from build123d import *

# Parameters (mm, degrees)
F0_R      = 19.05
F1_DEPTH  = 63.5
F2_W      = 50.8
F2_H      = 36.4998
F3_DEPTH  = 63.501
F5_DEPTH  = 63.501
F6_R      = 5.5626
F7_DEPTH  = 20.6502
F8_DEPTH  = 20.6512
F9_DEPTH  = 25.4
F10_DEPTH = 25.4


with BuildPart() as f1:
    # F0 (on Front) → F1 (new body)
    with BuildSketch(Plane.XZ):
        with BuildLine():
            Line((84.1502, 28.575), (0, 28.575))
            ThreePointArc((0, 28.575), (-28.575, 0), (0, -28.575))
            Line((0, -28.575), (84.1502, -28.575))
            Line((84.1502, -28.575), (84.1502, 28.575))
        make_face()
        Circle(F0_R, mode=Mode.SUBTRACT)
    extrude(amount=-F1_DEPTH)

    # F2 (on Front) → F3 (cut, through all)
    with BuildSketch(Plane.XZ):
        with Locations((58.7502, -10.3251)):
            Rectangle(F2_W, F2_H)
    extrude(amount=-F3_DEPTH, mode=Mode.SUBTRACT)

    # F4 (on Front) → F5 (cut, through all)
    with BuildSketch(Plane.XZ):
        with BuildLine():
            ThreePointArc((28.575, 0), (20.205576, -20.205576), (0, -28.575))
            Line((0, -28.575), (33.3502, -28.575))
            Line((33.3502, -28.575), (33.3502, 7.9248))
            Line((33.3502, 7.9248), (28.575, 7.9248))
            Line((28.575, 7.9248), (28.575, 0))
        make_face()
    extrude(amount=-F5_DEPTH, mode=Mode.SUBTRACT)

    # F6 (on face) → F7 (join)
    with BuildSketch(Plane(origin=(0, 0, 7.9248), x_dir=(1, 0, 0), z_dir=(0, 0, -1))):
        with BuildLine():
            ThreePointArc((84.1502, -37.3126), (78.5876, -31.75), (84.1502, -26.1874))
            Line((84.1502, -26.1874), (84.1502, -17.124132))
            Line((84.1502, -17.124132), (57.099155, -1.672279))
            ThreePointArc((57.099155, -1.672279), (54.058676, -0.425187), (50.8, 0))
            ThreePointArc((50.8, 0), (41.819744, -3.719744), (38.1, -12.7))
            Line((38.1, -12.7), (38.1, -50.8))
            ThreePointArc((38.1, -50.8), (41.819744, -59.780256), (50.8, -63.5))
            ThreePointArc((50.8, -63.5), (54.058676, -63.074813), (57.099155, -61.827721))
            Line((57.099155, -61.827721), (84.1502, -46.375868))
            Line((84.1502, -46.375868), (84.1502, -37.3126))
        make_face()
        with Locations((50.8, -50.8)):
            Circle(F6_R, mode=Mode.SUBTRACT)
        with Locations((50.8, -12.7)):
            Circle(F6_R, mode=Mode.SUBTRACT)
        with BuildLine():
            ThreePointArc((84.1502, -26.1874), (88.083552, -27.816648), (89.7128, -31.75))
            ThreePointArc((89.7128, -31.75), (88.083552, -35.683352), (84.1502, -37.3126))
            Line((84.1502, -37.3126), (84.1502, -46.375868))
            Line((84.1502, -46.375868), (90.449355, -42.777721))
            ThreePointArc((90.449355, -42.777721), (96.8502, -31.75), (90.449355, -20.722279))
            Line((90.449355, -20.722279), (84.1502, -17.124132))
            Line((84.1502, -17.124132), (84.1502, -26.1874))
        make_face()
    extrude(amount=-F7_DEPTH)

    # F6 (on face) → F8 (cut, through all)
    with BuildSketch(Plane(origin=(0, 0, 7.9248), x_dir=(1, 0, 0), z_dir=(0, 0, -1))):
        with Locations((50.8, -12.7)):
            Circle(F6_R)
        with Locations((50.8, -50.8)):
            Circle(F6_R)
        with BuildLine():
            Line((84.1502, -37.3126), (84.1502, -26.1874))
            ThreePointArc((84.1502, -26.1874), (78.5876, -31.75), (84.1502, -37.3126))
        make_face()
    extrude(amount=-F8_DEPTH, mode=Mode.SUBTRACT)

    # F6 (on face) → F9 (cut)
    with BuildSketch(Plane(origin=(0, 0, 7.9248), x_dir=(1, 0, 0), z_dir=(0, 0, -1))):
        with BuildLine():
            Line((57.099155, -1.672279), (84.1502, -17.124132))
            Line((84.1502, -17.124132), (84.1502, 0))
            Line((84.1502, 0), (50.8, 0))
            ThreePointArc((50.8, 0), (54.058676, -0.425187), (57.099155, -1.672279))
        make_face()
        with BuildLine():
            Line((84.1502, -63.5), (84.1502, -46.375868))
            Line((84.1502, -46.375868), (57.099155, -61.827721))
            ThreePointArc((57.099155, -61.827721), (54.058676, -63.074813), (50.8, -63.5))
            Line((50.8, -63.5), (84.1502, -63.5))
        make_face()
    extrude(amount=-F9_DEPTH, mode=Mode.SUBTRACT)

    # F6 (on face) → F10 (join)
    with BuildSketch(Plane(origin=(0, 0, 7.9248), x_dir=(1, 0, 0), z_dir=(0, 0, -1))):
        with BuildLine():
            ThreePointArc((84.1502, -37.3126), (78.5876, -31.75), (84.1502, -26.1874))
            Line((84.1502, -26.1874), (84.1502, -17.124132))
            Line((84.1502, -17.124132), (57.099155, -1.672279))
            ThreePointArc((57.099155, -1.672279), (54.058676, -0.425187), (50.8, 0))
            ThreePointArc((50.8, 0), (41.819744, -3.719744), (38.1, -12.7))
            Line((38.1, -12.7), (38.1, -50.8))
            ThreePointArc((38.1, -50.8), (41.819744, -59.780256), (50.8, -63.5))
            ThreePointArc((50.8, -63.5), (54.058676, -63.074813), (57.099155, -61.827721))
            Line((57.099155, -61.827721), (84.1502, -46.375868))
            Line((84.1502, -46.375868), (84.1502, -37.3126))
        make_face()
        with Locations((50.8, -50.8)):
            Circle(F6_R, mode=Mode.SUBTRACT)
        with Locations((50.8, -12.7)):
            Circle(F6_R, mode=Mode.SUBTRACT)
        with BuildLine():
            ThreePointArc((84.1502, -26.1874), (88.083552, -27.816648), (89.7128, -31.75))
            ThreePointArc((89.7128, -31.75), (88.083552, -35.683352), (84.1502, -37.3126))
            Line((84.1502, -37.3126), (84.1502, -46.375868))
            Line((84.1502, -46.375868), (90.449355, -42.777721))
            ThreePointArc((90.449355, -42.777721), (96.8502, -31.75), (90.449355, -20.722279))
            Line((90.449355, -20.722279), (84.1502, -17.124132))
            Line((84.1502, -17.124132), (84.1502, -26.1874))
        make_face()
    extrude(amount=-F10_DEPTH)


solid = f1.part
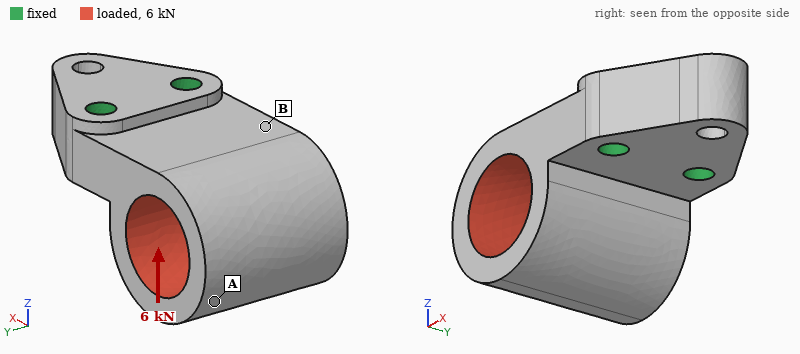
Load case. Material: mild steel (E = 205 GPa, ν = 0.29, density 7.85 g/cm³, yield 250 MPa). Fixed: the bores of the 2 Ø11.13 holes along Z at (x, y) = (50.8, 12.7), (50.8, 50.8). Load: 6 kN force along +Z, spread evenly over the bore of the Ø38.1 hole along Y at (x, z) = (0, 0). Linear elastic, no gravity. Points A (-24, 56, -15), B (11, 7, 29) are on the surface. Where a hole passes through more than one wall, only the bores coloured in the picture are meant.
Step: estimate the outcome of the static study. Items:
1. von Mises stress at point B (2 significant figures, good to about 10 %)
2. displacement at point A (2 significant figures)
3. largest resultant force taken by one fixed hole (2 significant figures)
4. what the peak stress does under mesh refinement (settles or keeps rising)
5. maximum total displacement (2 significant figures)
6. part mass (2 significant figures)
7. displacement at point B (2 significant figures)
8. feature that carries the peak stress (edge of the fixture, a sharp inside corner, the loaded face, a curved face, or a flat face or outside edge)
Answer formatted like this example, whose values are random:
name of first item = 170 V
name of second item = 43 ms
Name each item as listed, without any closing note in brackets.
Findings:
von Mises stress at point B = 30 MPa
displacement at point A = 59 µm
largest resultant force taken by one fixed hole = 3.0 kN
what the peak stress does under mesh refinement = keeps rising
maximum total displacement = 60 µm
part mass = 1.4 kg
displacement at point B = 17 µm
feature that carries the peak stress = edge of the fixture
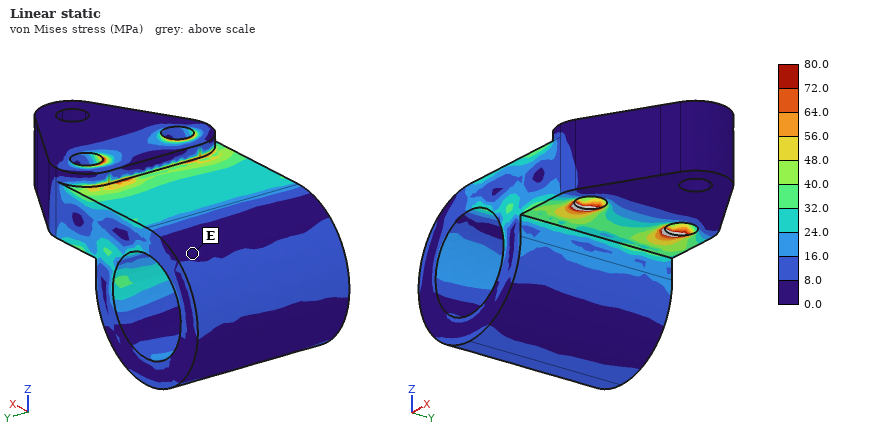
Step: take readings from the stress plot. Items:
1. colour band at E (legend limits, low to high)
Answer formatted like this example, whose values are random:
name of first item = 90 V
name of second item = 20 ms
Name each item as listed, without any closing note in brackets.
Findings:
colour band at E = 0.0 to 8.0 MPa
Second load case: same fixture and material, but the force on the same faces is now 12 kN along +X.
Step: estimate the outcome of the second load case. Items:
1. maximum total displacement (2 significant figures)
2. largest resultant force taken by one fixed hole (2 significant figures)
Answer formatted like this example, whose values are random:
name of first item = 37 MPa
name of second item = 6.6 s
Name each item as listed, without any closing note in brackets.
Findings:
maximum total displacement = 73 µm
largest resultant force taken by one fixed hole = 6.1 kN
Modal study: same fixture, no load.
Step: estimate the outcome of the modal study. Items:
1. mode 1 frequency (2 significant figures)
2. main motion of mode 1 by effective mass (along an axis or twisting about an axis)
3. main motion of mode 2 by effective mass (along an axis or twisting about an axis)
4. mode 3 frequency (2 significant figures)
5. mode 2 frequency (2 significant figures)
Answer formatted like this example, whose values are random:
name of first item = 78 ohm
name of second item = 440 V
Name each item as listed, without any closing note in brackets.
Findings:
mode 1 frequency = 2000 Hz
main motion of mode 1 by effective mass = along Z
main motion of mode 2 by effective mass = along Y
mode 3 frequency = 6700 Hz
mode 2 frequency = 4000 Hz
